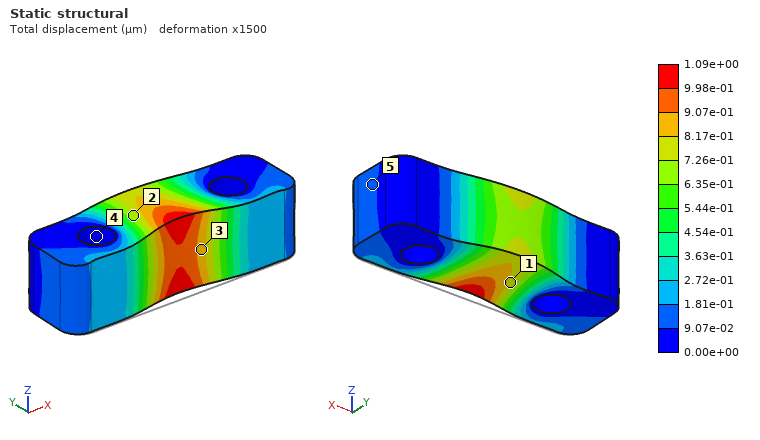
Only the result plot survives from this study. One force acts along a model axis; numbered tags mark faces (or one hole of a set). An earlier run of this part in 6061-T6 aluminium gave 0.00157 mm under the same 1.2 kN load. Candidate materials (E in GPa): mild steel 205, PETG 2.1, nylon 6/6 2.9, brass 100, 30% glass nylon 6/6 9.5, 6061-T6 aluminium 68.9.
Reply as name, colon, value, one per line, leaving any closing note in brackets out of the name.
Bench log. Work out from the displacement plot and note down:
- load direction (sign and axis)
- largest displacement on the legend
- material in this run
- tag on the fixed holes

load direction: +Y
largest displacement on the legend: 1.09e+00 µm
material in this run: brass
tag on the fixed holes: 4
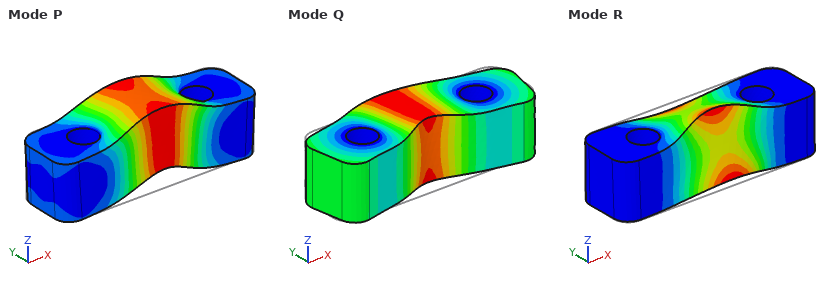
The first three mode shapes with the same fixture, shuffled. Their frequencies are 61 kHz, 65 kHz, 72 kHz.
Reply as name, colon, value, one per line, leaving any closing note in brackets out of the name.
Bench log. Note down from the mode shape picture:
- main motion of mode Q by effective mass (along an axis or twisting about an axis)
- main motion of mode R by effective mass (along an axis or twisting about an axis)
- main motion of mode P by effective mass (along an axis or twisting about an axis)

main motion of mode Q by effective mass: along Y
main motion of mode R by effective mass: twisting about X
main motion of mode P by effective mass: along Z
